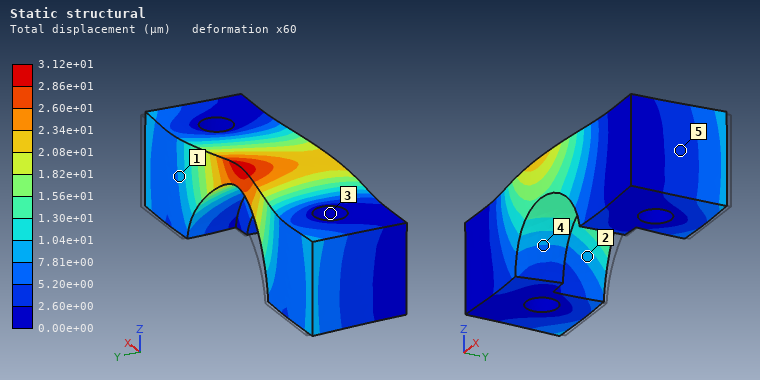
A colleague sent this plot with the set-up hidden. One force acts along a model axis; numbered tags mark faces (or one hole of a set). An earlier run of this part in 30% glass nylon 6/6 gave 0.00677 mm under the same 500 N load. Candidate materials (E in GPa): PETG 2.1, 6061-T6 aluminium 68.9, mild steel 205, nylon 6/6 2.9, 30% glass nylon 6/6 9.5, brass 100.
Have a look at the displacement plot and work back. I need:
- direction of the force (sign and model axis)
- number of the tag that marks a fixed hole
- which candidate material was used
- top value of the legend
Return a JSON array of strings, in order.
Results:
["-Y", "3", "PETG", "3.12e+01 µm"]
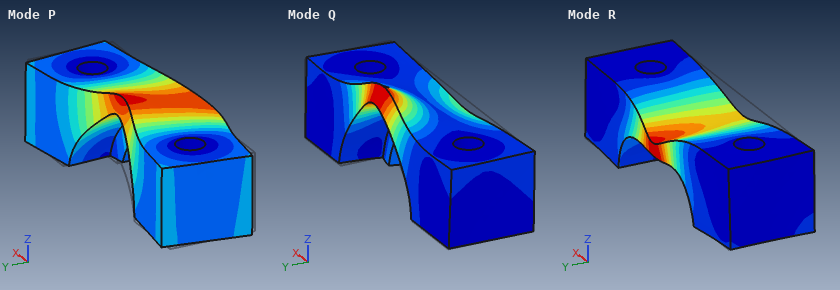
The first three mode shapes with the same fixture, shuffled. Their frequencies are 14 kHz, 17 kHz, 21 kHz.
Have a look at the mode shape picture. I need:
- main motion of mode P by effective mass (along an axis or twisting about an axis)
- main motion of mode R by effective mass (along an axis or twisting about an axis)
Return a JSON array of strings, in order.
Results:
["along Y", "along Z"]
